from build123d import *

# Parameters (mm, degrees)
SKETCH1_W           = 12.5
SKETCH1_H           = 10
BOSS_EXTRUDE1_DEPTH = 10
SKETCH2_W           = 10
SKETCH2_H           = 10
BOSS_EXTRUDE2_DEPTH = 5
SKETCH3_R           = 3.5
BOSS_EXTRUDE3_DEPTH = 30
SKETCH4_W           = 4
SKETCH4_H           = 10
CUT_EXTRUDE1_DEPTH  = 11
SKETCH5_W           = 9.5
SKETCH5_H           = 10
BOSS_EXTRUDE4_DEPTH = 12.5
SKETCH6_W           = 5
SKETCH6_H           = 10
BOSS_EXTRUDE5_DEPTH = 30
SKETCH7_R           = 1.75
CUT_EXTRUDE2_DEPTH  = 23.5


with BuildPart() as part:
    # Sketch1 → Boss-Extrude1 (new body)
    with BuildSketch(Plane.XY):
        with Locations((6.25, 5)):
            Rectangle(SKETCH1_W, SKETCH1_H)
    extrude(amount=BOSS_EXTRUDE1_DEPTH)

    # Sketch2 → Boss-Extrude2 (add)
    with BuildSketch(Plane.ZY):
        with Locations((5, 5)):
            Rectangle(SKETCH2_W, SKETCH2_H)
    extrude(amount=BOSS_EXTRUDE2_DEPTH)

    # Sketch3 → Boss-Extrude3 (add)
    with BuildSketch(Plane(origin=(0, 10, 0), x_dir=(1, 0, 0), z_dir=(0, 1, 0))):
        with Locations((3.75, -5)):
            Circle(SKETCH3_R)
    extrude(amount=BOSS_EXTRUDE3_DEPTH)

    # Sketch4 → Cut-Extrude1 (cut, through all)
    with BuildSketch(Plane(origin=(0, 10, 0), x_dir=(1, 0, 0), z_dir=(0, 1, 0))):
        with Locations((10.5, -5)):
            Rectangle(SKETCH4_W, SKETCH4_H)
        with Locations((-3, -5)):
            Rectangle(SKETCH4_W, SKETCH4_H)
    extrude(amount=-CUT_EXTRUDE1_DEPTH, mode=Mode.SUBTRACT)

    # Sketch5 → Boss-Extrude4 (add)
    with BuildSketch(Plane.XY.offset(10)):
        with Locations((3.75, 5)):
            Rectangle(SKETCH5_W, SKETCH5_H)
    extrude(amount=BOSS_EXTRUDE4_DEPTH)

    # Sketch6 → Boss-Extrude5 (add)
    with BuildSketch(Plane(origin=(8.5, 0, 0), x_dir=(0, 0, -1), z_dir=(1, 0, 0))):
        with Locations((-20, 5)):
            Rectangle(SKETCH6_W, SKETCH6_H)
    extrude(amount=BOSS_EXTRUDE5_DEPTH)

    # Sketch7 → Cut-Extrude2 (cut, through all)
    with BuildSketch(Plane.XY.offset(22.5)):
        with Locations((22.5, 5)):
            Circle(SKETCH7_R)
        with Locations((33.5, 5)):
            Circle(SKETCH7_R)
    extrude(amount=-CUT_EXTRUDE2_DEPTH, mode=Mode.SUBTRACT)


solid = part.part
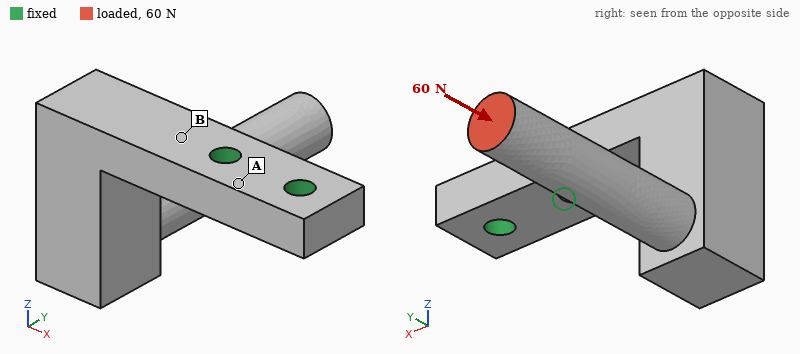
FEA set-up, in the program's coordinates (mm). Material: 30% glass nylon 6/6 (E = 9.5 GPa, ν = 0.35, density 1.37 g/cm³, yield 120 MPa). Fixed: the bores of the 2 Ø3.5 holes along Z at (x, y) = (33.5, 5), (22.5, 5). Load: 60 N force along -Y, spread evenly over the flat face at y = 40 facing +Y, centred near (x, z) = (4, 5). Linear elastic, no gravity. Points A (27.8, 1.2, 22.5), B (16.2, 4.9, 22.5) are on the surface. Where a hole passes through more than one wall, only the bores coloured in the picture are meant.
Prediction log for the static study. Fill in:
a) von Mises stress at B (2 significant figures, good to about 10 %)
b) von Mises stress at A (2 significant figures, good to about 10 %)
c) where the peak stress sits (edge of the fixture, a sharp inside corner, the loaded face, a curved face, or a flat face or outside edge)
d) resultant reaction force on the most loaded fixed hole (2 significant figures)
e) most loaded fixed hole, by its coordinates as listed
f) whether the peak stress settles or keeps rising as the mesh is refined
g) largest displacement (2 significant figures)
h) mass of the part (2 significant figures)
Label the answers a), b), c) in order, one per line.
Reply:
a) 19 MPa
b) 4.0 MPa
c) edge of the fixture
d) 100 N
e) (22.5, 5)
f) keeps rising
g) 0.55 mm
h) 6.4 g
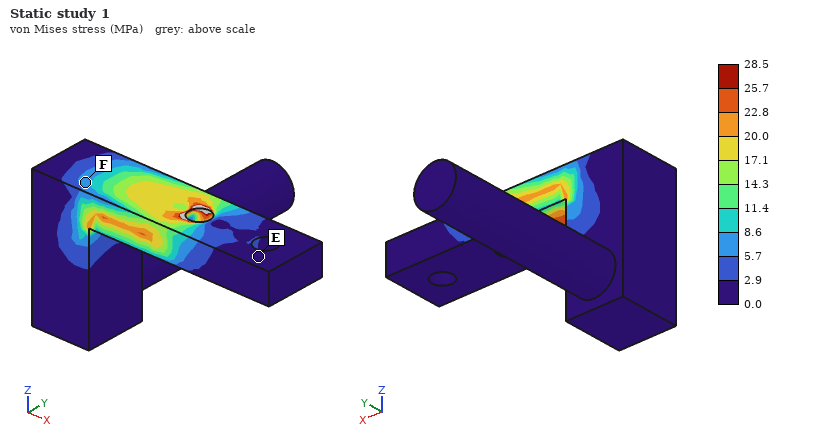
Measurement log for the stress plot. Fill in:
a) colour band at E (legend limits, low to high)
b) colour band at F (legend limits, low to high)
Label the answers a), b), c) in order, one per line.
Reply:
a) 0.0 to 2.9 MPa
b) 5.7 to 8.6 MPa
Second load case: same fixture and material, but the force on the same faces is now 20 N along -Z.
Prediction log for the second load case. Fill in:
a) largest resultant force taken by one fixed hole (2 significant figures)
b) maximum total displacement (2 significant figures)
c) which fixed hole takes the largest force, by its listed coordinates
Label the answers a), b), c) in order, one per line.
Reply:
a) 25 N
b) 0.66 mm
c) (22.5, 5)
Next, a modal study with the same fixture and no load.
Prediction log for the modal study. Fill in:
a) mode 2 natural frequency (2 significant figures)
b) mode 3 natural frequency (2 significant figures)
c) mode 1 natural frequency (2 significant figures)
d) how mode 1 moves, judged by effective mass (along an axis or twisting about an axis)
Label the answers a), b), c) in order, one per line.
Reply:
a) 1100 Hz
b) 2000 Hz
c) 930 Hz
d) along Z
